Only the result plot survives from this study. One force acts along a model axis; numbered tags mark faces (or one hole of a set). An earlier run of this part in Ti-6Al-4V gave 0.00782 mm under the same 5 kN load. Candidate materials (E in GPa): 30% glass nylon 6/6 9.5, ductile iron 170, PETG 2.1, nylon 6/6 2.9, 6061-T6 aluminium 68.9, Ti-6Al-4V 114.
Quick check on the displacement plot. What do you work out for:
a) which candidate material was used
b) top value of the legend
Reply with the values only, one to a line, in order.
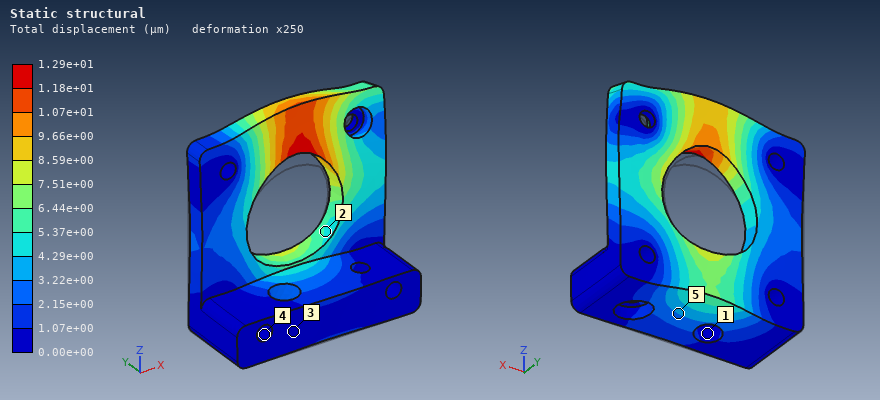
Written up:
6061-T6 aluminium
1.29e+01 µm
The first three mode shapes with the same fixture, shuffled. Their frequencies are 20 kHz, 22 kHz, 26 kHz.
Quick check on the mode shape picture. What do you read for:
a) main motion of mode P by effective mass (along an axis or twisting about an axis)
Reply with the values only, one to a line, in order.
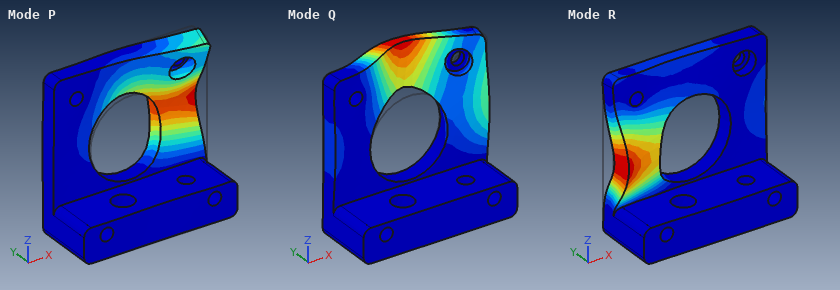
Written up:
along Y
